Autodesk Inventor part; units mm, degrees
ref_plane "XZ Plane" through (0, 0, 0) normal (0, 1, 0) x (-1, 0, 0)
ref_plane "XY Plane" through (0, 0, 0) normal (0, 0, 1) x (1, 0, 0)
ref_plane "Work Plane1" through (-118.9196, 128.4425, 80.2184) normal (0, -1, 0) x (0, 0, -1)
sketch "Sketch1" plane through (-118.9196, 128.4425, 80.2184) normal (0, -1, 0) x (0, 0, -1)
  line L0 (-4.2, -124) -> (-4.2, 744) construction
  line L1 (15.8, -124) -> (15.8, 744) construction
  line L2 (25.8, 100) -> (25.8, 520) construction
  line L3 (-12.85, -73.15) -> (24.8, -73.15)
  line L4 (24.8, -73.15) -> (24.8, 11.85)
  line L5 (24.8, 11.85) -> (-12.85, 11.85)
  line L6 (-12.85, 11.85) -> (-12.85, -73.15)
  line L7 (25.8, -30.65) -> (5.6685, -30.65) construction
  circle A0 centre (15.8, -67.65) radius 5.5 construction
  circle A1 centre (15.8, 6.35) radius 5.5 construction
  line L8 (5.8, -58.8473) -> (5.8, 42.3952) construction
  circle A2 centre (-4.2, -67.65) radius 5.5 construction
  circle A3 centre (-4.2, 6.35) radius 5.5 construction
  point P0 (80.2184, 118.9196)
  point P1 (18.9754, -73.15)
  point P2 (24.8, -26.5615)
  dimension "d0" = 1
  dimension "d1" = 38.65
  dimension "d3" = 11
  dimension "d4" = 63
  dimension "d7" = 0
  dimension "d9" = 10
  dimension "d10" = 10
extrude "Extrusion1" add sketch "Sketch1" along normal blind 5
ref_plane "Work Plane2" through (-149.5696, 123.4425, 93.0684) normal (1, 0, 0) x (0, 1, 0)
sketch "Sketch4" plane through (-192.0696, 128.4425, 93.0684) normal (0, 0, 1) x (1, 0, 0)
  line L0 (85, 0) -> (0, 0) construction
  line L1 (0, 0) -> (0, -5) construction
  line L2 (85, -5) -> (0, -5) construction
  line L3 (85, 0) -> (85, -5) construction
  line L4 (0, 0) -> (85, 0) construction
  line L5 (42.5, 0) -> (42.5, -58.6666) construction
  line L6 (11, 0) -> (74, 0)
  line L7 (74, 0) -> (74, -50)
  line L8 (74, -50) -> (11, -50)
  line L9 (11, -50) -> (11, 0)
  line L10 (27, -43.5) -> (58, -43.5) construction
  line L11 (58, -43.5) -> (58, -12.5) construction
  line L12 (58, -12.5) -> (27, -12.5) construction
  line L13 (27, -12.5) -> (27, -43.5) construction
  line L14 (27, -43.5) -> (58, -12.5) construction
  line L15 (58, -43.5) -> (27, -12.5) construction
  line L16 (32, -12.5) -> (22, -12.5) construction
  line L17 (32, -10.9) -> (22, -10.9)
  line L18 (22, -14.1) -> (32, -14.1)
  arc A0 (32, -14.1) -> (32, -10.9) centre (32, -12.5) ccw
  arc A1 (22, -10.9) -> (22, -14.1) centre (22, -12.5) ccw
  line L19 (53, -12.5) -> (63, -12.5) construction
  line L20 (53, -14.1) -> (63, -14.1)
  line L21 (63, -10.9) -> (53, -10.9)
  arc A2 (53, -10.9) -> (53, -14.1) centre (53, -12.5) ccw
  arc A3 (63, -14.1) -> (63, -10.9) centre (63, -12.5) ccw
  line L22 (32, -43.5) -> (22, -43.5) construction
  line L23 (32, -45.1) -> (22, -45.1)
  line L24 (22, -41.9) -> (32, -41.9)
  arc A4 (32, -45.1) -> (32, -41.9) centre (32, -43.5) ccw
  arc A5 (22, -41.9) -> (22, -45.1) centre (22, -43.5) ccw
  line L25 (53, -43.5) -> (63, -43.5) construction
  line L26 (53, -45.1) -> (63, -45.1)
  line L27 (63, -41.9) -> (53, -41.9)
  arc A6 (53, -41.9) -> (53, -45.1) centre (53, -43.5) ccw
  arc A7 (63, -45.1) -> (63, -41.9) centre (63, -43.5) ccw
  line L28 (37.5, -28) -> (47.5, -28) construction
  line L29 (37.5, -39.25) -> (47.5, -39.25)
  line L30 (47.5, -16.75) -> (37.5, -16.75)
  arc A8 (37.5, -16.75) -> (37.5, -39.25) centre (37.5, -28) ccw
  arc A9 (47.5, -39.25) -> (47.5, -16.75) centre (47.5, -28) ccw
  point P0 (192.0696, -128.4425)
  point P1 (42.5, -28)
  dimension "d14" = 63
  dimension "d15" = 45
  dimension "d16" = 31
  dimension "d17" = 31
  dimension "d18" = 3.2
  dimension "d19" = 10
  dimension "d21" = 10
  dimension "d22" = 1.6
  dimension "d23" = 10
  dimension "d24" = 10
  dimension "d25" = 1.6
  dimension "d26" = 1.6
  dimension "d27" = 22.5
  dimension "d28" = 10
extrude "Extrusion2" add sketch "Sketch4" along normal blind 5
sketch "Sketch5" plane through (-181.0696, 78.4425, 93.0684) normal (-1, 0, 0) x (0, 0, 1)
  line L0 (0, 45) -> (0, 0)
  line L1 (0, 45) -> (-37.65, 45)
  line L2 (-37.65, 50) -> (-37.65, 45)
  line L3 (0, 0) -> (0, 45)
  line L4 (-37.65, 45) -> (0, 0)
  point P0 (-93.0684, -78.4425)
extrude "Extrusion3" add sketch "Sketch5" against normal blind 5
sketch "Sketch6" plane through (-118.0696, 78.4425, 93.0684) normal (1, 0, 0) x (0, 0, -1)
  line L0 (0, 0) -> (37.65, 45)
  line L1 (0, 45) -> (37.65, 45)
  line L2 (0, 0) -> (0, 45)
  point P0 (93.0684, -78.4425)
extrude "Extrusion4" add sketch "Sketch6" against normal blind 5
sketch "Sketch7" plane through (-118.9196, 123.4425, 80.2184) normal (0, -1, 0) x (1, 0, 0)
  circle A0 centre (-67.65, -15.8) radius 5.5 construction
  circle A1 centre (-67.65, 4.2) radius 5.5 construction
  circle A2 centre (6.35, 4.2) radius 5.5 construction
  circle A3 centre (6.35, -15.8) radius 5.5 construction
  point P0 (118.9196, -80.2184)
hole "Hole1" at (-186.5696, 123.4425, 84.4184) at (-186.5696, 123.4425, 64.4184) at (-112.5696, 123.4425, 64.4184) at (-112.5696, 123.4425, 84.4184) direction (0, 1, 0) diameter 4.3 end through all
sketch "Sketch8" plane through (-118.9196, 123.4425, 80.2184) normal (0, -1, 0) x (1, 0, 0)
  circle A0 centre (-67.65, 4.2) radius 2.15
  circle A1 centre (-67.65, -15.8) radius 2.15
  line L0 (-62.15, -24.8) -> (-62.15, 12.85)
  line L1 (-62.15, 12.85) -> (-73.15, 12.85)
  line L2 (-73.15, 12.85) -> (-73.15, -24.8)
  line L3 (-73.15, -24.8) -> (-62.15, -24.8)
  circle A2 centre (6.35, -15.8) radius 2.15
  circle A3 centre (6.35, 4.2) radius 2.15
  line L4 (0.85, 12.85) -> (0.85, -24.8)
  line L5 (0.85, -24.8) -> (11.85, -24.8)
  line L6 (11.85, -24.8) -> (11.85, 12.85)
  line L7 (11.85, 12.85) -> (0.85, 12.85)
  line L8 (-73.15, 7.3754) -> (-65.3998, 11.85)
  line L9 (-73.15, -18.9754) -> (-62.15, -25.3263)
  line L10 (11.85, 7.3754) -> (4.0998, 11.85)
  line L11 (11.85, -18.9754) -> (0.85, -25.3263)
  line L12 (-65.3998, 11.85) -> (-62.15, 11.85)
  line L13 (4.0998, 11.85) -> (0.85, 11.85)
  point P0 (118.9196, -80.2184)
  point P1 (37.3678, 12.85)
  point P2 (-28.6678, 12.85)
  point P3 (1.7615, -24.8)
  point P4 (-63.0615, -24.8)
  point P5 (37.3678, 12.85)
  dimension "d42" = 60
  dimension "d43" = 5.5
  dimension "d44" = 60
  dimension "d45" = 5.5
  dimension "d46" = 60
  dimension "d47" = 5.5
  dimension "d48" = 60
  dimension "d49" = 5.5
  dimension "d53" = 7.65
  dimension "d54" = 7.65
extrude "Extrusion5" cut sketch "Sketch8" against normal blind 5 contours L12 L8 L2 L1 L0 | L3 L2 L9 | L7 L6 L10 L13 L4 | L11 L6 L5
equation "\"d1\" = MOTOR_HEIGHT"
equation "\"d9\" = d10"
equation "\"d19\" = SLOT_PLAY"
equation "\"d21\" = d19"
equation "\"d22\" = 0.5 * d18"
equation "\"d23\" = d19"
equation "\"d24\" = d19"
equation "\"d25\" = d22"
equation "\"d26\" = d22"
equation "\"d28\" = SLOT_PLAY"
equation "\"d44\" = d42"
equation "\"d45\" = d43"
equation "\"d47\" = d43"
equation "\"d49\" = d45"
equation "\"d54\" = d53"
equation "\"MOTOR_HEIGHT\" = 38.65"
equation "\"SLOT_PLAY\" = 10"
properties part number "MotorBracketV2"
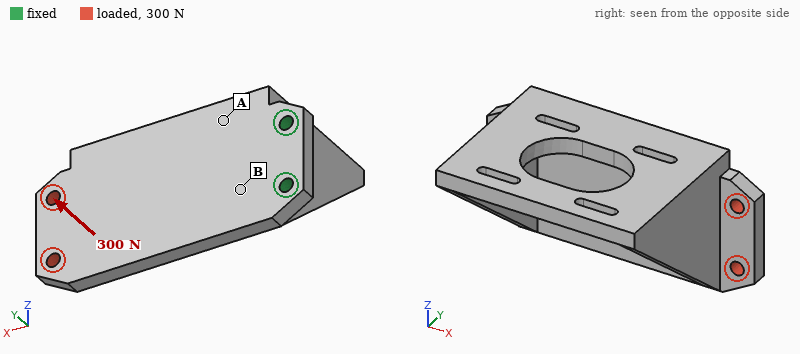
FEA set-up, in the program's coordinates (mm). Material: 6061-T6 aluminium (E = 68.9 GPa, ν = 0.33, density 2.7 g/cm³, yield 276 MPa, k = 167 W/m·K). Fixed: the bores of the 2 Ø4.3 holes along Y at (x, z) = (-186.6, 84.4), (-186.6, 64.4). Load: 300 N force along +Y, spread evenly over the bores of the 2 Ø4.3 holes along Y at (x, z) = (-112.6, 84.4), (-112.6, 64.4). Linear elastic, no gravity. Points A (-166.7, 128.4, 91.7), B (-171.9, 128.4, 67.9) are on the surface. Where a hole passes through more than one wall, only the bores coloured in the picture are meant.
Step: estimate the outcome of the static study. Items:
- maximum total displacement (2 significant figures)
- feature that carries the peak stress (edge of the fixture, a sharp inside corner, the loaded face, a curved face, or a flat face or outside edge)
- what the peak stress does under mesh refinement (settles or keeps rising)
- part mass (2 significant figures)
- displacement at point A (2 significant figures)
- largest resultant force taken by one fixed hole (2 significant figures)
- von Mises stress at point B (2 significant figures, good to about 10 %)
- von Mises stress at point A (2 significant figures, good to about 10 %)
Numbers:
0.78 mm
edge of the fixture
keeps rising
96 g
0.14 mm
170 N
51 MPa
22 MPa
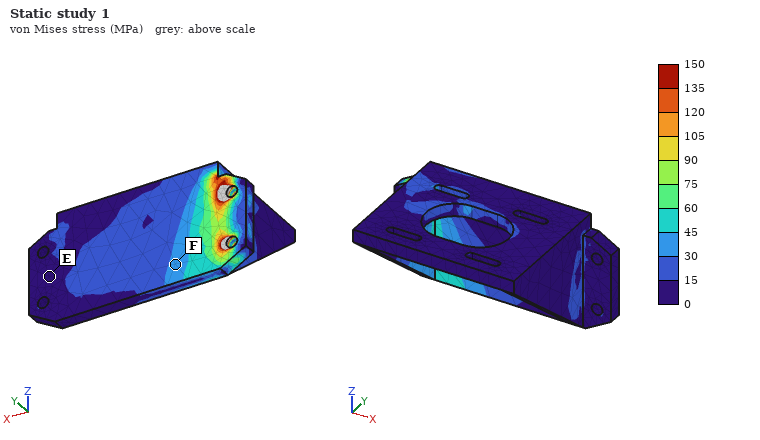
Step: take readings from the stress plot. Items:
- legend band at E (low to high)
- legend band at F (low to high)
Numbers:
0 to 15 MPa
30 to 45 MPa
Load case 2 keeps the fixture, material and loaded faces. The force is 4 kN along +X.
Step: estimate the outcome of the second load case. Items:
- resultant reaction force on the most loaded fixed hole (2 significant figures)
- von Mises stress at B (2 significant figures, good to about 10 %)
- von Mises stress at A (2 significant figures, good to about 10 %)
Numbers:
2.0 kN
24 MPa
14 MPa
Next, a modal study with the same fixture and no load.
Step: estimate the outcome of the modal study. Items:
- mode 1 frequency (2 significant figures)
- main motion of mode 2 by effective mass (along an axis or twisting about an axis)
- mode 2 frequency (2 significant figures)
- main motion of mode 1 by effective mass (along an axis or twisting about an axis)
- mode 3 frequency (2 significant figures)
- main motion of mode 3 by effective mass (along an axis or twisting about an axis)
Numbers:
550 Hz
along Z
1500 Hz
along Y
3000 Hz
along Z
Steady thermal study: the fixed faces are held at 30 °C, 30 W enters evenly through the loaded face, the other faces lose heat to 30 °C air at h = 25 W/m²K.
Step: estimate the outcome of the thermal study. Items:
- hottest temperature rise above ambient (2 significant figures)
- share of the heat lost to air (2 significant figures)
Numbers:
47 K
27 %
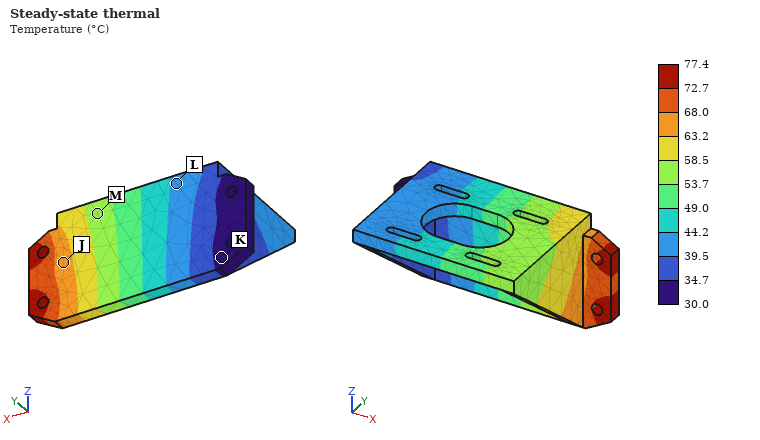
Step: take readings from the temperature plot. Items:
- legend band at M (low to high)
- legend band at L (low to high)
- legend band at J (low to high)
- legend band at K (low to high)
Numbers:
53.7 to 58.5 °C
39.5 to 44.2 °C
63.2 to 68.0 °C
30.0 to 34.7 °C
